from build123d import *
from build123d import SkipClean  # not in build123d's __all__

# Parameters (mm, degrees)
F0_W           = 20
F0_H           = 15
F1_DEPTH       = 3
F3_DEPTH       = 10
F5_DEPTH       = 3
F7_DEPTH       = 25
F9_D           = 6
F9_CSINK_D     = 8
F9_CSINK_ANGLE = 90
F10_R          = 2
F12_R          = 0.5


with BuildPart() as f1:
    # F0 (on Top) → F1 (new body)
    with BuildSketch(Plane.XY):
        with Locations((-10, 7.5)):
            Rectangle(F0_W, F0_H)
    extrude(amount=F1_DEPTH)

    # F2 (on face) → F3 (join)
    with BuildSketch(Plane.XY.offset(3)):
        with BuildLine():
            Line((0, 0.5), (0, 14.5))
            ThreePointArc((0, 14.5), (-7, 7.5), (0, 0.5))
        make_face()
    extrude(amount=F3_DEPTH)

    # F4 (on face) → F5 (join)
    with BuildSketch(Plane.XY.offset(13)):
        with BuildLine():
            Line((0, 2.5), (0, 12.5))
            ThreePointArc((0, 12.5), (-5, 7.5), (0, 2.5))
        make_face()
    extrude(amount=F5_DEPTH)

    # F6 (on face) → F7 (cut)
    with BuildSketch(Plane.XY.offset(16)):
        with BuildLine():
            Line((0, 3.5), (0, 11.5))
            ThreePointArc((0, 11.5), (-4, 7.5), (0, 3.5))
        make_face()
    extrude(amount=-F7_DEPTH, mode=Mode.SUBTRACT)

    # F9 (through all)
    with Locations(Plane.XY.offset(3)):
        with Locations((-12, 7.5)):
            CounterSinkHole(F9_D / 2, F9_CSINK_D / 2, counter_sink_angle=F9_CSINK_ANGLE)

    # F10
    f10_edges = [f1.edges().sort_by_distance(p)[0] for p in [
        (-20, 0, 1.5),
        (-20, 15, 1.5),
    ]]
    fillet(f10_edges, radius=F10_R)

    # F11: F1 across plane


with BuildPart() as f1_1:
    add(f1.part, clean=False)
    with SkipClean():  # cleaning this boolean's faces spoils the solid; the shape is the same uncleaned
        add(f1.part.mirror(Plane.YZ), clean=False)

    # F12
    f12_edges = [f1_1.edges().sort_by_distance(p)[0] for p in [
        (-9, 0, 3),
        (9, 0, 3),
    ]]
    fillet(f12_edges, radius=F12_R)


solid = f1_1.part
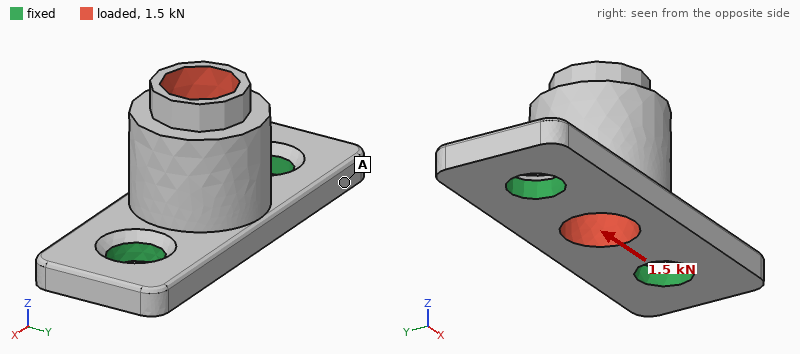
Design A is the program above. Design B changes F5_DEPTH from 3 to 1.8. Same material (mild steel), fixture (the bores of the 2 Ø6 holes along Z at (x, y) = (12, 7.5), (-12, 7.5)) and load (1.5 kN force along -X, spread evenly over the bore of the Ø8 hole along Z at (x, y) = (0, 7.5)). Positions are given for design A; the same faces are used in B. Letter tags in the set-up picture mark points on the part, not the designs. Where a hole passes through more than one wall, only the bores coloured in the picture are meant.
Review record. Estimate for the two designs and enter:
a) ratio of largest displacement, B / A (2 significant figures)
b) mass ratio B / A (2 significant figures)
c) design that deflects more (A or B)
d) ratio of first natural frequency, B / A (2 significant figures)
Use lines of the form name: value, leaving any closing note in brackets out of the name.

ratio of largest displacement, B / A: 0.82
mass ratio B / A: 0.99
design that deflects more: A
ratio of first natural frequency, B / A: 1.0
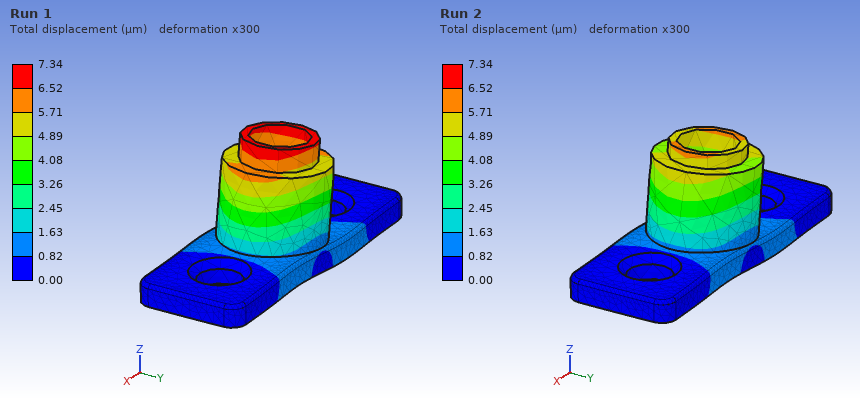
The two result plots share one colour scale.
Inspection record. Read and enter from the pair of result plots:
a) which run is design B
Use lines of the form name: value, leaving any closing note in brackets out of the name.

which run is design B: Run 2
